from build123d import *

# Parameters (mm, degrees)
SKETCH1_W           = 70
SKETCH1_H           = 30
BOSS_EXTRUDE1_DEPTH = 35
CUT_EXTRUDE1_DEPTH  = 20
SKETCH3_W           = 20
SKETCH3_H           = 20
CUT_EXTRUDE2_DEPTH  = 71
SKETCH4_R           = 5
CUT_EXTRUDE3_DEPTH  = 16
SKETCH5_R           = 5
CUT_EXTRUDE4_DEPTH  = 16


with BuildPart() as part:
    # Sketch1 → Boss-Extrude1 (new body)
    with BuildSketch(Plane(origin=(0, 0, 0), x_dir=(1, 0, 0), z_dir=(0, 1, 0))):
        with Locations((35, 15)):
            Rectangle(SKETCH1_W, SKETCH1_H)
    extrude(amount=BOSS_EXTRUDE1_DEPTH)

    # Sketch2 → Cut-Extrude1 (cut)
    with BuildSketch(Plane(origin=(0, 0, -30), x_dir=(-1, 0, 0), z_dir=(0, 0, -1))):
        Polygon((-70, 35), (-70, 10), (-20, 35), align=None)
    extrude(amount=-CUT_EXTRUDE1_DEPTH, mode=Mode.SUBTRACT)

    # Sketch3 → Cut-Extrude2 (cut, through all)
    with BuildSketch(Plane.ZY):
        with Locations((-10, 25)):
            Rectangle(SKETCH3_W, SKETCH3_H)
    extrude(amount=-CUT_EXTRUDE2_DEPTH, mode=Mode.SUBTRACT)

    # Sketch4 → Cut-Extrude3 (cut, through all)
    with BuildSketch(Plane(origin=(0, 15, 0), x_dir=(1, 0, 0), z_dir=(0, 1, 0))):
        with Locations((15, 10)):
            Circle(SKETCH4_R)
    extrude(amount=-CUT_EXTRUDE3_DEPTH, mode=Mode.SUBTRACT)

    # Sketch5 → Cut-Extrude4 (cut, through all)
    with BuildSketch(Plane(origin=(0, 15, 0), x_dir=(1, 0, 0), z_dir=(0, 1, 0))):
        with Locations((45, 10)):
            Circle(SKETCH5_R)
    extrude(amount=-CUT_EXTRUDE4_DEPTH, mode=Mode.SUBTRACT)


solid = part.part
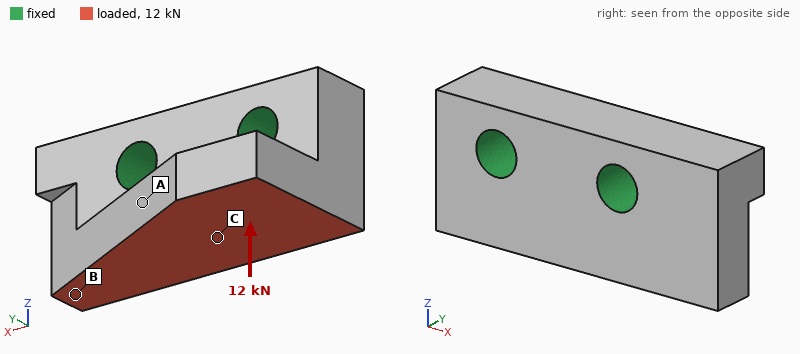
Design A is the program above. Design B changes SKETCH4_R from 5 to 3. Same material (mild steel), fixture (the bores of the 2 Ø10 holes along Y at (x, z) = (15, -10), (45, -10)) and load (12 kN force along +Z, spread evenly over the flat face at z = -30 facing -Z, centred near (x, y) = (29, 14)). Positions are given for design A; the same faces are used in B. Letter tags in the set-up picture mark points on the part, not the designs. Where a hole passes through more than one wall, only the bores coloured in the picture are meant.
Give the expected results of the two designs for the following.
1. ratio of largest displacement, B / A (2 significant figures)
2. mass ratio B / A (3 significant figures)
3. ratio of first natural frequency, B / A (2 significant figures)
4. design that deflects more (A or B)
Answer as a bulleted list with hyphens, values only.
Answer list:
- 1.1
- 1.02
- 0.92
- B
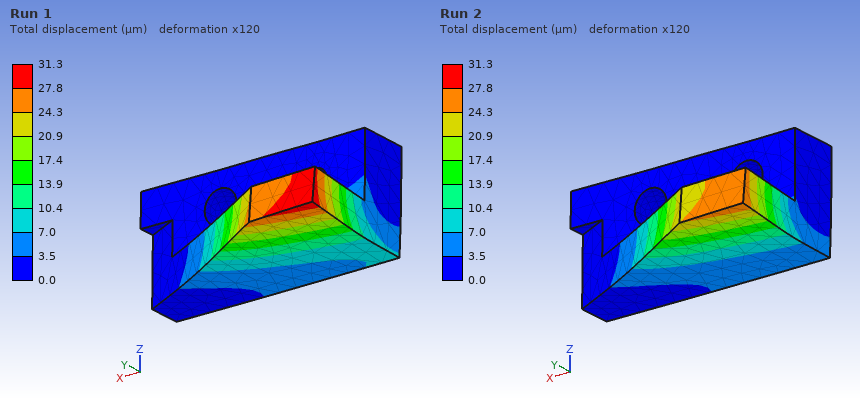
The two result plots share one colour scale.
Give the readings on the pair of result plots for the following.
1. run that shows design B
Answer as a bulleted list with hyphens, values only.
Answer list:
- Run 1
